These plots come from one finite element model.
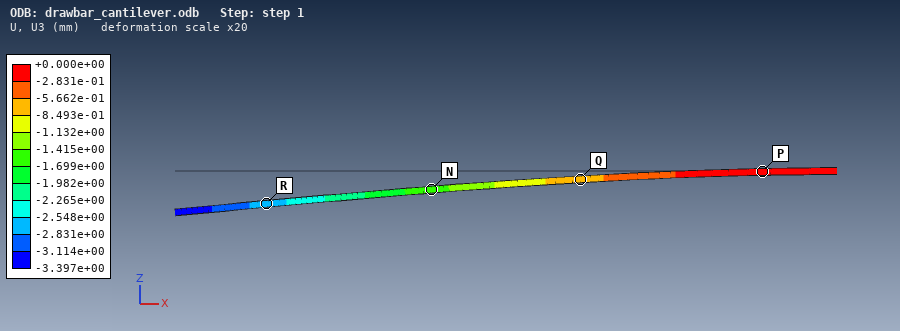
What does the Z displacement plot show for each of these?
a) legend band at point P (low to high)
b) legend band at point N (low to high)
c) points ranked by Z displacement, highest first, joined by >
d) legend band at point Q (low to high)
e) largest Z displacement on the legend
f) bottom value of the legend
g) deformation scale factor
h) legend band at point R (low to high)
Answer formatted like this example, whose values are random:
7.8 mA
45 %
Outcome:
-2.831e-01 to +0.000e+00 mm
-1.699e+00 to -1.415e+00 mm
P > Q > N > R
-8.493e-01 to -5.662e-01 mm
+0.000e+00 mm
-3.397e+00 mm
20
-2.831e+00 to -2.548e+00 mm
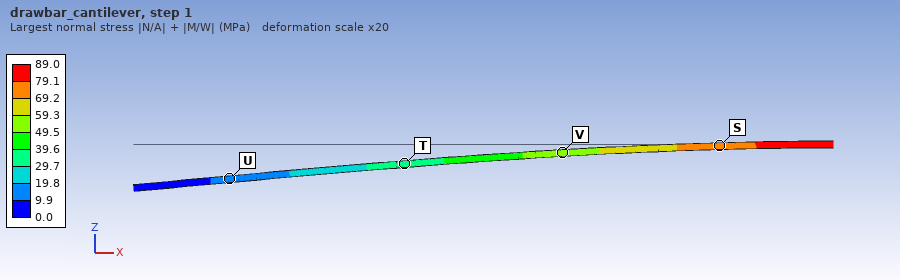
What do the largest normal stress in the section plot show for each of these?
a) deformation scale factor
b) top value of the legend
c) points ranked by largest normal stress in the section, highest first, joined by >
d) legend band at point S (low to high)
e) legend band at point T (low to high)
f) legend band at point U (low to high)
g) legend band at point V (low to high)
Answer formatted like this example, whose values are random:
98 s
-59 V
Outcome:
20
89.0 MPa
S > V > T > U
69.2 to 79.1 MPa
29.7 to 39.6 MPa
9.9 to 19.8 MPa
49.5 to 59.3 MPa
